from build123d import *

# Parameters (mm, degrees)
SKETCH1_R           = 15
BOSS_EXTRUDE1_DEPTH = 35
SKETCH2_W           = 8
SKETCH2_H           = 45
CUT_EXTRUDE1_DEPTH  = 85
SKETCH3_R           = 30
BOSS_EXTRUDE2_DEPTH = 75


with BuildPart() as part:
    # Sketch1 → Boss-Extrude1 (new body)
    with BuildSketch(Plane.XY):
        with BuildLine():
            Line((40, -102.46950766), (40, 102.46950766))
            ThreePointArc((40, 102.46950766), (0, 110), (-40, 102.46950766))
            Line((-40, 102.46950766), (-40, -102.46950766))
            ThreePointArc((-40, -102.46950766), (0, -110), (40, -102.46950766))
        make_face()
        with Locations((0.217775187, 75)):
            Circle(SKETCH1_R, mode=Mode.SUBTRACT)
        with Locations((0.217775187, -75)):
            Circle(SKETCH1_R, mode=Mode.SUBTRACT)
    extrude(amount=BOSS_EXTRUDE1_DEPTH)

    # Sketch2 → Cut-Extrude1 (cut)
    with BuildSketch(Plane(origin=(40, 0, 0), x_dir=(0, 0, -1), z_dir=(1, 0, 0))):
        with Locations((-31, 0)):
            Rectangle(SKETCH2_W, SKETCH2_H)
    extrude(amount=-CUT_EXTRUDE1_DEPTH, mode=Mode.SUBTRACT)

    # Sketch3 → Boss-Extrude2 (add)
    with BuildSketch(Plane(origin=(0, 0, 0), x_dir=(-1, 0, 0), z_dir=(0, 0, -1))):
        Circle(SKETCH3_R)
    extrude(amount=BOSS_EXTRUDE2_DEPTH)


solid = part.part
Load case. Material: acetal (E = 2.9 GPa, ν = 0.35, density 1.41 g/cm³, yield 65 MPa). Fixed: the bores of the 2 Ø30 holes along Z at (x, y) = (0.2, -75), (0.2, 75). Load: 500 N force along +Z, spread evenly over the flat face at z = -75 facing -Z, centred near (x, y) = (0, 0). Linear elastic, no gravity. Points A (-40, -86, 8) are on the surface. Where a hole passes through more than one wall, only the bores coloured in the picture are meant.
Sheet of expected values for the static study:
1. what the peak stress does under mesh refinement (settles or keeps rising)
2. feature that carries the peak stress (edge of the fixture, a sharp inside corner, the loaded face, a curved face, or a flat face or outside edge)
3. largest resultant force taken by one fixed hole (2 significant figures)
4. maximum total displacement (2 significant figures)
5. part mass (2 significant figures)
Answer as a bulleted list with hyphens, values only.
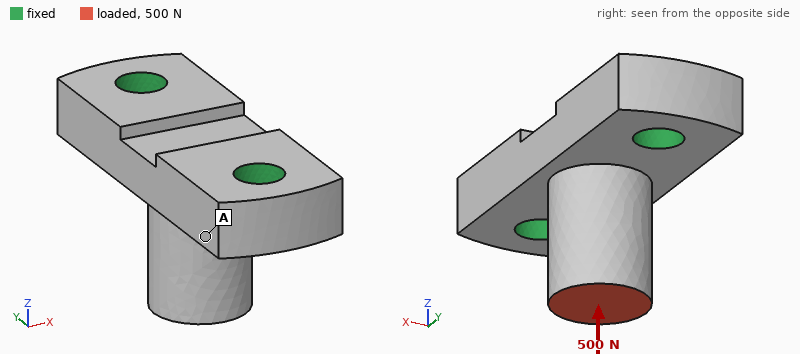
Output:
- keeps rising
- edge of the fixture
- 280 N
- 15 µm
- 1.0 kg
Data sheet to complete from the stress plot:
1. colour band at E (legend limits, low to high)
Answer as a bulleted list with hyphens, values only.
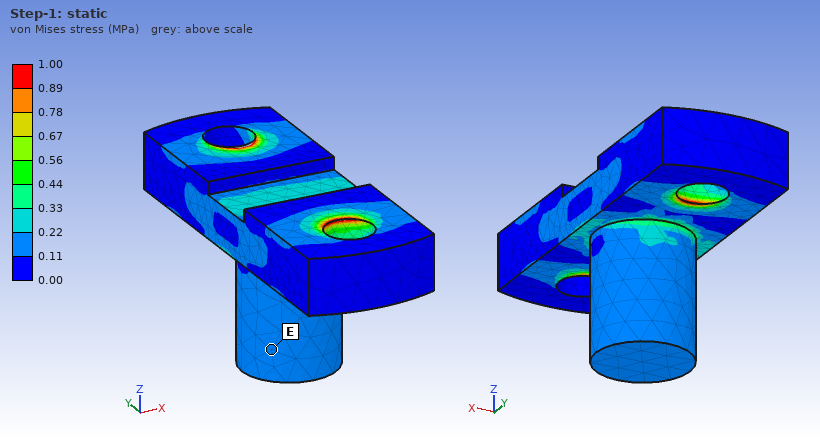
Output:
- 0.11 to 0.22 MPa
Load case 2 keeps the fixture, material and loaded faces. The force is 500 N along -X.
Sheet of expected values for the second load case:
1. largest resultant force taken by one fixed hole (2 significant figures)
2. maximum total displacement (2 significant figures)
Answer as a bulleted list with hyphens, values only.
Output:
- 250 N
- 0.20 mm
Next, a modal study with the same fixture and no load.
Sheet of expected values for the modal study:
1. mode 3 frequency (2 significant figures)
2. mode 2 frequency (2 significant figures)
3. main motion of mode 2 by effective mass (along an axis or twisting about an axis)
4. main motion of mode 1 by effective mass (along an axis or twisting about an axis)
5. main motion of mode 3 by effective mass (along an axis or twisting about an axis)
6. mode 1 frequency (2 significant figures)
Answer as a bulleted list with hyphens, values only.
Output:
- 1500 Hz
- 1100 Hz
- along Y
- along X
- along Z
- 720 Hz
